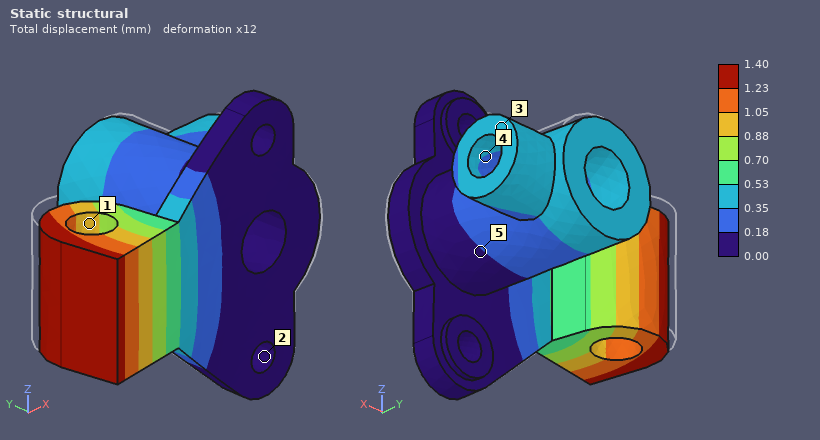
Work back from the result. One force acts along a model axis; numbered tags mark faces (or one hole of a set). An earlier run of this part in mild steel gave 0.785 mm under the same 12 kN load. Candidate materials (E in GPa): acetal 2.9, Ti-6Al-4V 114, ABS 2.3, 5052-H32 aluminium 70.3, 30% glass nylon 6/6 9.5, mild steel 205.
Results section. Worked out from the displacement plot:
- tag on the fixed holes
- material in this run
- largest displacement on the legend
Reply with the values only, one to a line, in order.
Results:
2
Ti-6Al-4V
1.40 mm
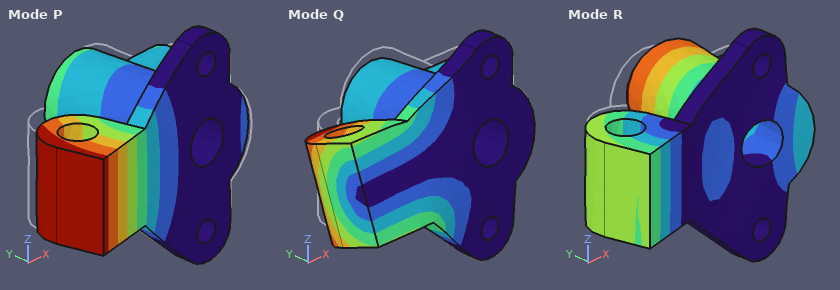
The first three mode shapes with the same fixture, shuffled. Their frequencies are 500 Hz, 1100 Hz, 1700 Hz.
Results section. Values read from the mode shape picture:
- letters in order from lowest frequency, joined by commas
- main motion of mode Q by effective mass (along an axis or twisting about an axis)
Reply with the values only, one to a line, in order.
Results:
P, R, Q
along Z
